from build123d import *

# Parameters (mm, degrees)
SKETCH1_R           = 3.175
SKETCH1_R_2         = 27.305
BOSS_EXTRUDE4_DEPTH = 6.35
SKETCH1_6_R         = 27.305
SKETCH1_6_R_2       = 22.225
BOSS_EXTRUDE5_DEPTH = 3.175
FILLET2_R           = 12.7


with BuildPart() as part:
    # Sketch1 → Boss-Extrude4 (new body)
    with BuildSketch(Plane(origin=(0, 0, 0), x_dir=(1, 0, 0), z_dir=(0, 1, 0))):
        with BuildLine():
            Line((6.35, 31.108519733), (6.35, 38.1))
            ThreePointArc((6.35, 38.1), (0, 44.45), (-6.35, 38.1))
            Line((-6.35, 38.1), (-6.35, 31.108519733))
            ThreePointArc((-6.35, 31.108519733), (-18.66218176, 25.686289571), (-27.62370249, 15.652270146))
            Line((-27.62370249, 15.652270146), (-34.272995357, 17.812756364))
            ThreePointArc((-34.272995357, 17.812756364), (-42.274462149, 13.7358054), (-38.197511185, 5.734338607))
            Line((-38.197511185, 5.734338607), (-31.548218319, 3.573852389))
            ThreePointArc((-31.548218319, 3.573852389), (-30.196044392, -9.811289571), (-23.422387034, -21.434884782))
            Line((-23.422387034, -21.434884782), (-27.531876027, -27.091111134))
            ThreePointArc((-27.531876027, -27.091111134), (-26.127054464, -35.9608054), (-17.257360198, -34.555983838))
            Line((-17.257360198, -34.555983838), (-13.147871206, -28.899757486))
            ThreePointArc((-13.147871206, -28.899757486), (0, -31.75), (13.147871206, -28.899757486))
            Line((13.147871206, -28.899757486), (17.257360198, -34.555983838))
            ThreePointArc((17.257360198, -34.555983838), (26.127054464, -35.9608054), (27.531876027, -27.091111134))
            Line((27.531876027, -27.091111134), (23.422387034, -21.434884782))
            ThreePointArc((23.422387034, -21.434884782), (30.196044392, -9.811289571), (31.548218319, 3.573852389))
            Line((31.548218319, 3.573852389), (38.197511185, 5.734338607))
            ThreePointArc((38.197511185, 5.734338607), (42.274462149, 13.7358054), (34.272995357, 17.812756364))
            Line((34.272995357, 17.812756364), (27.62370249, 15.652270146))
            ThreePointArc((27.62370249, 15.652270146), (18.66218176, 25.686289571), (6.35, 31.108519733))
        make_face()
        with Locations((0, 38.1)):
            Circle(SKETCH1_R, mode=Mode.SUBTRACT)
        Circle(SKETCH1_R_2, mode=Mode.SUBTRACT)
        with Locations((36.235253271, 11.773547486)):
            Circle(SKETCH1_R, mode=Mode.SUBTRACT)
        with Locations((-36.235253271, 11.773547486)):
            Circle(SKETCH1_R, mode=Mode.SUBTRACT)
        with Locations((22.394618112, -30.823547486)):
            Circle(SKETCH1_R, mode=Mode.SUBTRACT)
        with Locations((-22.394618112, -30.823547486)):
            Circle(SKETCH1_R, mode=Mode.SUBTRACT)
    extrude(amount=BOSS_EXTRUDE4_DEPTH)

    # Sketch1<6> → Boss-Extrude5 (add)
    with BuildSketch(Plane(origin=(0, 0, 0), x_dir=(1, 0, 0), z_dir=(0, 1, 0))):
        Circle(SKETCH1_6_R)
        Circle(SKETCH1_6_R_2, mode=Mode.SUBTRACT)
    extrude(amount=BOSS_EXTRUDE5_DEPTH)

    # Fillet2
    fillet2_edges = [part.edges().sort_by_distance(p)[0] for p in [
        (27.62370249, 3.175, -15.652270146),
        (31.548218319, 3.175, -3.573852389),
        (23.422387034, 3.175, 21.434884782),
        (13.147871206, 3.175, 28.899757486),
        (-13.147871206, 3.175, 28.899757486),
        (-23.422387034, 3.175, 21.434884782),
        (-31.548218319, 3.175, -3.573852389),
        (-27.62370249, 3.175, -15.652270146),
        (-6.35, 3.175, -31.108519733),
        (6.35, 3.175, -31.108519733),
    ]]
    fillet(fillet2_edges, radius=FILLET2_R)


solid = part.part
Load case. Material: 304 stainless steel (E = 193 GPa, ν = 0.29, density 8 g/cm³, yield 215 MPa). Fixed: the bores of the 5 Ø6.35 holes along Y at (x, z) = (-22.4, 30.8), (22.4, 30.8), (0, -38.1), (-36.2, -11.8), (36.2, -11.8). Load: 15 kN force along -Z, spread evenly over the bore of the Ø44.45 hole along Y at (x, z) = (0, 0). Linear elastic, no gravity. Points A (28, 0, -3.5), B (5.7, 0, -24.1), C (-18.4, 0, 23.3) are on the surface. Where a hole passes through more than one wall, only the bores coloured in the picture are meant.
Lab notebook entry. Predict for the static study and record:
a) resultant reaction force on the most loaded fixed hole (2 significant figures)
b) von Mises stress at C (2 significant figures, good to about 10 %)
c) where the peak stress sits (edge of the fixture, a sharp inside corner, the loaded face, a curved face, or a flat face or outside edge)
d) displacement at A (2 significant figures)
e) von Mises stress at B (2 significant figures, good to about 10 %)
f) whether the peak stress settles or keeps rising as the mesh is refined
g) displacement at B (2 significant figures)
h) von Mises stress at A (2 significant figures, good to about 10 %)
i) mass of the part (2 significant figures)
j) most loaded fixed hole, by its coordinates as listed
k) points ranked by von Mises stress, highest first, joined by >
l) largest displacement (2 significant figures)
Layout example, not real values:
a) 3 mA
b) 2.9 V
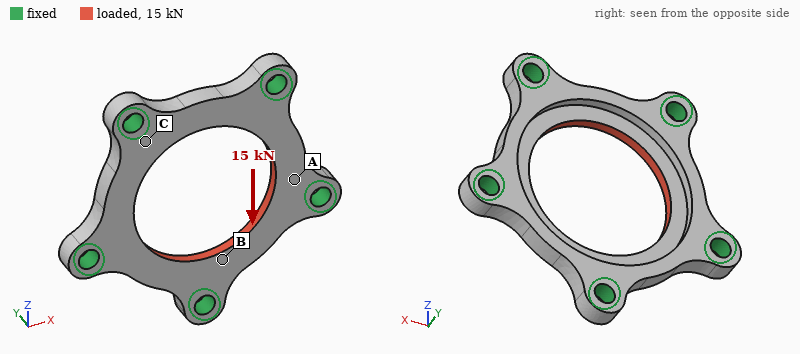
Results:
a) 4.0 kN
b) 52 MPa
c) edge of the fixture
d) 4.3 µm
e) 77 MPa
f) keeps rising
g) 6.7 µm
h) 17 MPa
i) 98 g
j) (0, -38.1)
k) B > C > A
l) 15 µm
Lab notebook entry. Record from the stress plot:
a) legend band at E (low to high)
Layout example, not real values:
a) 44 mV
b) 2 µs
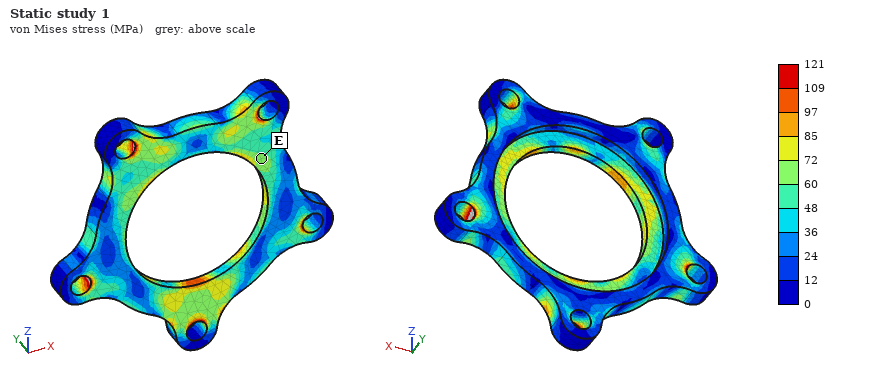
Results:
a) 60 to 72 MPa
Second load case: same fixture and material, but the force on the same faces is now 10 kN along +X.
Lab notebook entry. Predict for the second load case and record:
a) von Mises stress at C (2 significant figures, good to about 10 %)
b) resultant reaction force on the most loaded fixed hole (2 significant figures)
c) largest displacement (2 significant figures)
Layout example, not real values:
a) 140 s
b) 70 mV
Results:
a) 31 MPa
b) 2.6 kN
c) 9.5 µm
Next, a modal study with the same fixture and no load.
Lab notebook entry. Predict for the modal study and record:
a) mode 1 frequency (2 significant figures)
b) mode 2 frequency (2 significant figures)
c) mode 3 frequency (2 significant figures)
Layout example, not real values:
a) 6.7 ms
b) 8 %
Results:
a) 17 kHz
b) 17 kHz
c) 17 kHz
